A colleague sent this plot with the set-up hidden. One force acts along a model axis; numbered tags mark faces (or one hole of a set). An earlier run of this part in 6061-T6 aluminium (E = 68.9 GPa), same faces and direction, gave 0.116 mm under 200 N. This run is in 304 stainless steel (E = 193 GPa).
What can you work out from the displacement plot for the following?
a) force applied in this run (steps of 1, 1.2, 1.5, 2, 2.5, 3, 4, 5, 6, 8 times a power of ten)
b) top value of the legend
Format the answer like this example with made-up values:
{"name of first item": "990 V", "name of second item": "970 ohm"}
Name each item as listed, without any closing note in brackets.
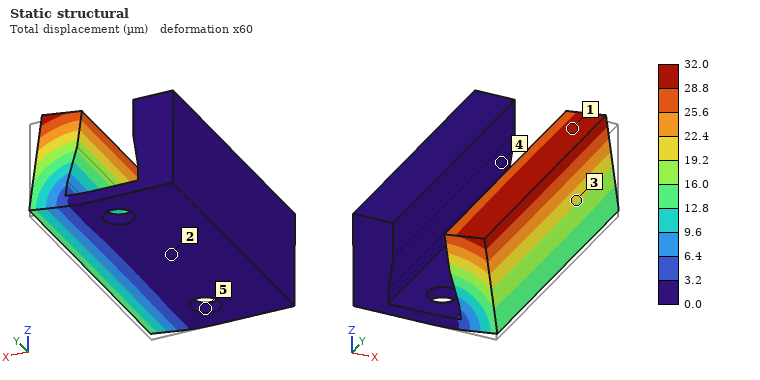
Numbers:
{"force applied in this run": "150 N", "top value of the legend": "32.0 µm"}
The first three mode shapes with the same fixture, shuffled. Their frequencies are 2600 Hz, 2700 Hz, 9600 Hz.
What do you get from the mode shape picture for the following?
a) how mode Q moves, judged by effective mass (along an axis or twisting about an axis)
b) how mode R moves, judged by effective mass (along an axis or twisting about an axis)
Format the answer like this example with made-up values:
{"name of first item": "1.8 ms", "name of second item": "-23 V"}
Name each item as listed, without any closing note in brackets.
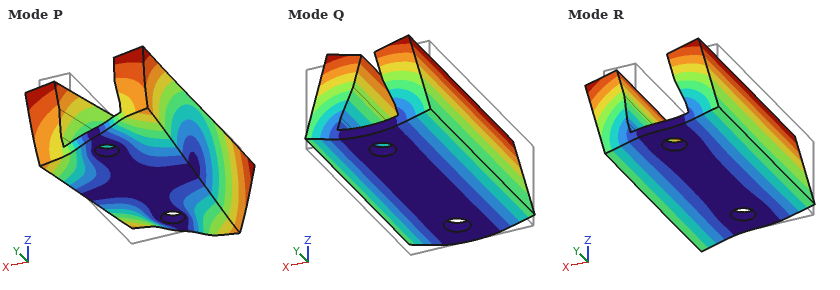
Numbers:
{"how mode Q moves, judged by effective mass": "along Z", "how mode R moves, judged by effective mass": "along X"}
